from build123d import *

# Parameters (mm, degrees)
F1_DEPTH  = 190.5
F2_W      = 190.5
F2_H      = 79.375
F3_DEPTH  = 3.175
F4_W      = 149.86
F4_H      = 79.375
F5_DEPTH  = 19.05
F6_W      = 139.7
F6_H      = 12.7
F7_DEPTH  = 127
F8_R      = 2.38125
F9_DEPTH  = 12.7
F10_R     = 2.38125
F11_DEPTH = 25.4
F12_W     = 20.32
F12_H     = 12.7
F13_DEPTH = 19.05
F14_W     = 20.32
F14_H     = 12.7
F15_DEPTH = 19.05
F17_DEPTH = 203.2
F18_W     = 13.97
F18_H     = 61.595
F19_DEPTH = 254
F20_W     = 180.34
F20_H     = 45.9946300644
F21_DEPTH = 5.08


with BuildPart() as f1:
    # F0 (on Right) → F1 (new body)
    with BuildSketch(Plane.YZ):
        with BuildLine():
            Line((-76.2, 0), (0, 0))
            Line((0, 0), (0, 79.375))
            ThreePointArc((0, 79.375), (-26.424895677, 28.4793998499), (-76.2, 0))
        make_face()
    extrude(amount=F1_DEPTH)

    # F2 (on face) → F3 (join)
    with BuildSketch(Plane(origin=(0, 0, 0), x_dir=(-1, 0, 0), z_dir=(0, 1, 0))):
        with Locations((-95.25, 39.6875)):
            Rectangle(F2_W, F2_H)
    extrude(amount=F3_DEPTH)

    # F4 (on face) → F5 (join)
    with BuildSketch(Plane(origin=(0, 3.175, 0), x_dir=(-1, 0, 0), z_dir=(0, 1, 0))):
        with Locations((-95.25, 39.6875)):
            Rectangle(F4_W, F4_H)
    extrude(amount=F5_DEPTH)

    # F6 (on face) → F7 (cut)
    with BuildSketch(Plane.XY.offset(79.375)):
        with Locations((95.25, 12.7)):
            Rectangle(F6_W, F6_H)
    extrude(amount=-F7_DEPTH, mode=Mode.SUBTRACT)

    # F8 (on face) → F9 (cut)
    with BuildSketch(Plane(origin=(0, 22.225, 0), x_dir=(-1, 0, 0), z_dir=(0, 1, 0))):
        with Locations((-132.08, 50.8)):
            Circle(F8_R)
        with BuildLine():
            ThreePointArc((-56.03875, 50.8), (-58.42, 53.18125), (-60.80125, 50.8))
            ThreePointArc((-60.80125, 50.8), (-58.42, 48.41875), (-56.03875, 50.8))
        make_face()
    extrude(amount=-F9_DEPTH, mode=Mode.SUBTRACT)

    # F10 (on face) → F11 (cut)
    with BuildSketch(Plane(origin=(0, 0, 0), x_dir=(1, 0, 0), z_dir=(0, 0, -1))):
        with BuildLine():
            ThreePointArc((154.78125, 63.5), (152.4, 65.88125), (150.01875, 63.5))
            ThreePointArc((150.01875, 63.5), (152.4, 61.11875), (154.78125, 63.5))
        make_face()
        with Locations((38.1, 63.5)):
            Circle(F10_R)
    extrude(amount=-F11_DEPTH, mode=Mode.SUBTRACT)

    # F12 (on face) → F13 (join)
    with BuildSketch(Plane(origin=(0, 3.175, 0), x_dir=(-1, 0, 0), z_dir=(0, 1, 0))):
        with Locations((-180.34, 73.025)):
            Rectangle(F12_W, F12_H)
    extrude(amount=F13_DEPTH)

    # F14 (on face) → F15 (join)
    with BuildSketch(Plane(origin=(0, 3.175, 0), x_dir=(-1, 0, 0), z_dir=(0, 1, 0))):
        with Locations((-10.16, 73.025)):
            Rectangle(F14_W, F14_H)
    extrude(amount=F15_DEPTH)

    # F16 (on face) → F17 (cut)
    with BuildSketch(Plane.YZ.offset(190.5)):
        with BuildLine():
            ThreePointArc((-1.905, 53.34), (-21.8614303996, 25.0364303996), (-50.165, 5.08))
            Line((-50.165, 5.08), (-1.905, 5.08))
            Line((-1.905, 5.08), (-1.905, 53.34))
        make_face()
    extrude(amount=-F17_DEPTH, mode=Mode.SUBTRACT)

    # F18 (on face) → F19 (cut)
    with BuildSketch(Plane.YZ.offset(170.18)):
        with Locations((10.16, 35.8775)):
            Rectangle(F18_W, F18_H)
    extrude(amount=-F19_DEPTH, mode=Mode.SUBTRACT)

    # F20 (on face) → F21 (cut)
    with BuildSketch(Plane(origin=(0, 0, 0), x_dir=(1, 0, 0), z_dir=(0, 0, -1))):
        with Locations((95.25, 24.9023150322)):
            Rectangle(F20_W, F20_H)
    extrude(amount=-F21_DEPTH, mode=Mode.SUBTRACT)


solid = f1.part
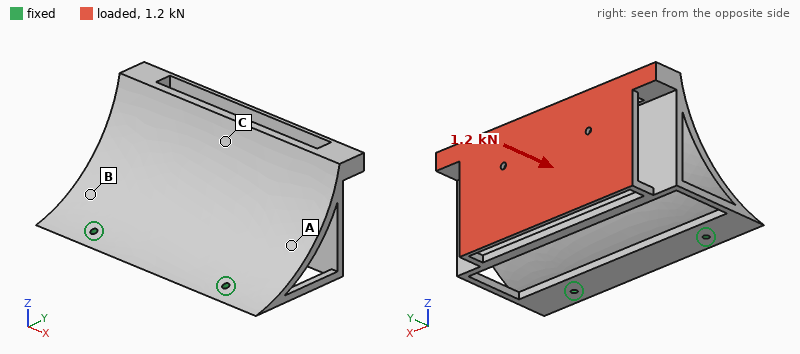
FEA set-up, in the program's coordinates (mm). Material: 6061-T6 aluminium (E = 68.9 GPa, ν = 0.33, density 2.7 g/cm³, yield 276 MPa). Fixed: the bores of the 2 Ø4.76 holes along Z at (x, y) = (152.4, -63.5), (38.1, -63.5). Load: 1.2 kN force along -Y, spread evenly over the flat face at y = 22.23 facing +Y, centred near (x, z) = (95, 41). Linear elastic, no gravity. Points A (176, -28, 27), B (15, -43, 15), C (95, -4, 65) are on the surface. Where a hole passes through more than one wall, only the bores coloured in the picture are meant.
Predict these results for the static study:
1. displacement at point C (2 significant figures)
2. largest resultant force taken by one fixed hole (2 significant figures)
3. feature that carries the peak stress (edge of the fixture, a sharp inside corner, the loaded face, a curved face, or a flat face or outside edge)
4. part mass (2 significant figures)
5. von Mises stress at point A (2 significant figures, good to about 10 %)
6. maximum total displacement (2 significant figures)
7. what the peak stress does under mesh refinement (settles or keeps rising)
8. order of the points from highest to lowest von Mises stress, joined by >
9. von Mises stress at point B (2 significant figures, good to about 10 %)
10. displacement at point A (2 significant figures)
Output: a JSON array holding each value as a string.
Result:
["1.5 mm", "600 N", "edge of the fixture", "650 g", "24 MPa", "2.7 mm", "keeps rising", "B > A > C", "43 MPa", "0.62 mm"]
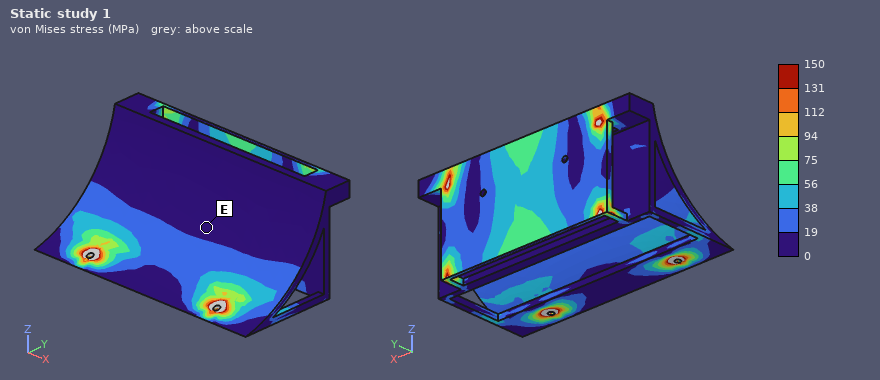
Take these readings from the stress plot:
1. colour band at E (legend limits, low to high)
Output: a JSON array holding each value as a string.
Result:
["0 to 19 MPa"]
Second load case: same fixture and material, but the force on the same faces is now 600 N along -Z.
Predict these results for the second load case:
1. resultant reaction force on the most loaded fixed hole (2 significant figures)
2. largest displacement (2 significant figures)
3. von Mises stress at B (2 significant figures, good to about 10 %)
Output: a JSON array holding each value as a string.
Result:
["440 N", "2.2 mm", "41 MPa"]
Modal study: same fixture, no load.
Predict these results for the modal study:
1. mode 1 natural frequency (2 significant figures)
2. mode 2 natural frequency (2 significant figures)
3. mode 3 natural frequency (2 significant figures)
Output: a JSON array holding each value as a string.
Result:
["150 Hz", "460 Hz", "670 Hz"]
